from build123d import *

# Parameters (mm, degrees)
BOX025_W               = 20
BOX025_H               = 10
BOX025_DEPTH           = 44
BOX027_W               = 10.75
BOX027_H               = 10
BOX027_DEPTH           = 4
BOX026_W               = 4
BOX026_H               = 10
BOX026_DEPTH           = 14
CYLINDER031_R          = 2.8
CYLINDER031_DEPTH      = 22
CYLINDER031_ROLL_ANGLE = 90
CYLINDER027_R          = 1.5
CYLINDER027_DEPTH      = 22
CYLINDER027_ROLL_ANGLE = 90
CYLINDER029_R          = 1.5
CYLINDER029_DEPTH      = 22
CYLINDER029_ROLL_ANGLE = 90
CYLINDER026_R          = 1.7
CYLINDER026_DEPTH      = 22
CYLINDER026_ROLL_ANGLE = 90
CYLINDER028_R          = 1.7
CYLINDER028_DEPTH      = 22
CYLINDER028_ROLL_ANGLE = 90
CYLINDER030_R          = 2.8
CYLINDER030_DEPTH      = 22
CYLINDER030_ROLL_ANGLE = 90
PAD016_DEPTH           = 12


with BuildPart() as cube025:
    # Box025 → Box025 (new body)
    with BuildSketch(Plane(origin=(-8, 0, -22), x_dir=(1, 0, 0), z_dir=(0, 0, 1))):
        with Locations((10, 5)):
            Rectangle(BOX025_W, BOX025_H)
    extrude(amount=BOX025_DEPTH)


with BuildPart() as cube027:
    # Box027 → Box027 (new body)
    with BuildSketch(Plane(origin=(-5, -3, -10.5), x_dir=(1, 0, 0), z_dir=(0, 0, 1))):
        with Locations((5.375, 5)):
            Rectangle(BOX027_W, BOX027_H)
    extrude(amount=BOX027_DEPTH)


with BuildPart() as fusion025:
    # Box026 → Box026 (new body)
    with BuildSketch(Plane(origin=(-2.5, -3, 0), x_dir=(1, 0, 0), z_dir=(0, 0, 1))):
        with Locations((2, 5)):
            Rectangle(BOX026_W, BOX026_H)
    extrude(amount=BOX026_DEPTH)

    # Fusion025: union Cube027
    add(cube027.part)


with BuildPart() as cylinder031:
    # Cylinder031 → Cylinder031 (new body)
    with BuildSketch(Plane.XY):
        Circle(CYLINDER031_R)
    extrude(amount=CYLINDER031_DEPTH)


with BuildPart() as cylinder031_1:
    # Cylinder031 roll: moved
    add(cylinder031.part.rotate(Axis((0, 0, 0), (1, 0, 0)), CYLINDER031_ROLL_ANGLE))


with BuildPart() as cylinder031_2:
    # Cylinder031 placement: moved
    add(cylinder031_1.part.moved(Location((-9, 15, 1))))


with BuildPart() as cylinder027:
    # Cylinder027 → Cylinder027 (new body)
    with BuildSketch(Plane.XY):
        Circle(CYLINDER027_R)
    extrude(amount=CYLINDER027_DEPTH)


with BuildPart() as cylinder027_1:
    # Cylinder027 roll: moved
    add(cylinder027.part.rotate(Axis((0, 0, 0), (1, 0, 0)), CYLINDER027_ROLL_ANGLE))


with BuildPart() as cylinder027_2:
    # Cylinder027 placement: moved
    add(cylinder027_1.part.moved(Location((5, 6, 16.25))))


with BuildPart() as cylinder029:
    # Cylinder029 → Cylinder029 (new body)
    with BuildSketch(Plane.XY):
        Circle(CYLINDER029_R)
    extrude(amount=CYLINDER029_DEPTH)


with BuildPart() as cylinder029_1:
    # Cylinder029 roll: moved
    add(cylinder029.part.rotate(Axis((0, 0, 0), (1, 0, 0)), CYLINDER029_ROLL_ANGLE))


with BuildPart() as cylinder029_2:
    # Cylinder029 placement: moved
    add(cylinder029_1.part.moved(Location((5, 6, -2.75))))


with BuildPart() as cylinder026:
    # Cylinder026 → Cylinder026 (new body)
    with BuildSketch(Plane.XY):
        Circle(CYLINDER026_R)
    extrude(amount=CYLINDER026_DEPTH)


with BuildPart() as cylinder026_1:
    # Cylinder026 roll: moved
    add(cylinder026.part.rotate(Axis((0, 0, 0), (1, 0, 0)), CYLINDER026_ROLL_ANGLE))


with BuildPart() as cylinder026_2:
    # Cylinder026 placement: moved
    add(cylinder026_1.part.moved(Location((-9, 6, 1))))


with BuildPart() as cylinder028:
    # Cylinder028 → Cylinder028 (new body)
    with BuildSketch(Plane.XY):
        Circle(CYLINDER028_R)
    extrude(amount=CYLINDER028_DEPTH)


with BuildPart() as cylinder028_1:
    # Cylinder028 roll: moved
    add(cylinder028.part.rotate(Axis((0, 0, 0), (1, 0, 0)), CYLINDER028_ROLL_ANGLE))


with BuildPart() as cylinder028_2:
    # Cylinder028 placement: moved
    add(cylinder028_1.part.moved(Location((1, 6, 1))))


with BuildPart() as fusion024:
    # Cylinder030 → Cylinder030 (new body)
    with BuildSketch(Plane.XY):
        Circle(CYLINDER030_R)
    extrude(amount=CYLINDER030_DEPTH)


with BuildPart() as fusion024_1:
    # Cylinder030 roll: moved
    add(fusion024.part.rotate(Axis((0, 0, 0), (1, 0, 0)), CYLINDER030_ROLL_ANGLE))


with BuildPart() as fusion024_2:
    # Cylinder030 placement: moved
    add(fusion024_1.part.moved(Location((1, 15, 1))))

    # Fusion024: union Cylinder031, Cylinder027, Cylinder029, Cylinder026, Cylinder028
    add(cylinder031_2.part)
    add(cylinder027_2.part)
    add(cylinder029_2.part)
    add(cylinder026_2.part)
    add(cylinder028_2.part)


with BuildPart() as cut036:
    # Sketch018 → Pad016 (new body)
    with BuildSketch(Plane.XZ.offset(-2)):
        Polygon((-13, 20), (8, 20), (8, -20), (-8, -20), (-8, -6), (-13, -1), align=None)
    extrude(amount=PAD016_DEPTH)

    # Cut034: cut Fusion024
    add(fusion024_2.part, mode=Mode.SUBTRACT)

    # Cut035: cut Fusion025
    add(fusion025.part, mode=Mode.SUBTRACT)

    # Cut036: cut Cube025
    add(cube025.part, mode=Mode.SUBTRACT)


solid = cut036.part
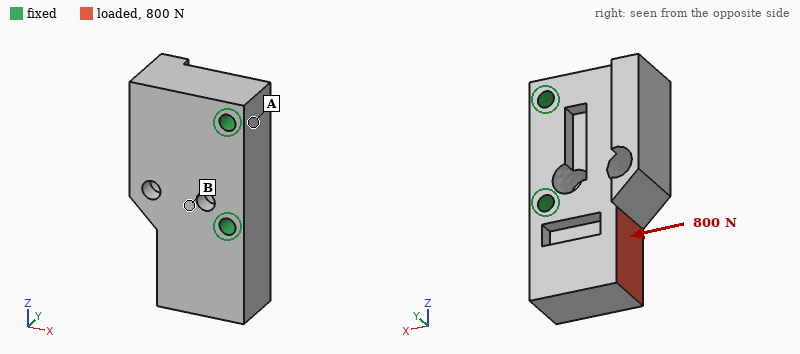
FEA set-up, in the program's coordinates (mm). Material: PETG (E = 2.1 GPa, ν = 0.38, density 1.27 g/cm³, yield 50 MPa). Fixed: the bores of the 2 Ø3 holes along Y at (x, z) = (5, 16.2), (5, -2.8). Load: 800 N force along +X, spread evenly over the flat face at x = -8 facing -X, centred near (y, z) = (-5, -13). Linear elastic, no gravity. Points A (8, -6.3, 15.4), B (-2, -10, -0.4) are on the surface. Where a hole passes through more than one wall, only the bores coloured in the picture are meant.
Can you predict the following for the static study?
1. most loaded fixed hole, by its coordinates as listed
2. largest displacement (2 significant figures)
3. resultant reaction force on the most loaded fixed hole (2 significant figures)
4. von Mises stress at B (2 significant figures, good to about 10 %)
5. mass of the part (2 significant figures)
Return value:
(5, -2.8)
0.43 mm
1.1 kN
13 MPa
8.9 g
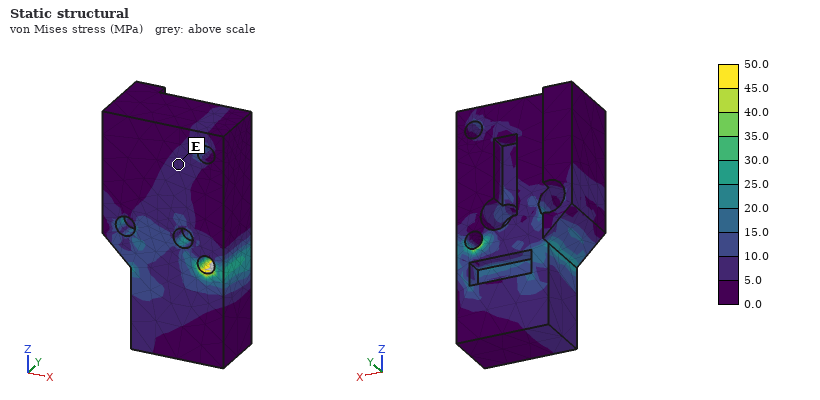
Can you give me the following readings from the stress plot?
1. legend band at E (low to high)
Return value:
5.0 to 10.0 MPa
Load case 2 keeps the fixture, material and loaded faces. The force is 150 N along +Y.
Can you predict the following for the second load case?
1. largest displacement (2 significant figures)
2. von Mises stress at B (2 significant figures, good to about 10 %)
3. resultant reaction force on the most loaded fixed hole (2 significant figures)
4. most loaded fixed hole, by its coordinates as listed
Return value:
0.25 mm
4.5 MPa
170 N
(5, -2.8)
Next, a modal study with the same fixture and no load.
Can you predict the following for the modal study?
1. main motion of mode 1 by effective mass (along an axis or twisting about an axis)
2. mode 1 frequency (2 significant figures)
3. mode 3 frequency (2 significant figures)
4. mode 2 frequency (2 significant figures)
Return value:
along Y
3800 Hz
4500 Hz
4200 Hz
